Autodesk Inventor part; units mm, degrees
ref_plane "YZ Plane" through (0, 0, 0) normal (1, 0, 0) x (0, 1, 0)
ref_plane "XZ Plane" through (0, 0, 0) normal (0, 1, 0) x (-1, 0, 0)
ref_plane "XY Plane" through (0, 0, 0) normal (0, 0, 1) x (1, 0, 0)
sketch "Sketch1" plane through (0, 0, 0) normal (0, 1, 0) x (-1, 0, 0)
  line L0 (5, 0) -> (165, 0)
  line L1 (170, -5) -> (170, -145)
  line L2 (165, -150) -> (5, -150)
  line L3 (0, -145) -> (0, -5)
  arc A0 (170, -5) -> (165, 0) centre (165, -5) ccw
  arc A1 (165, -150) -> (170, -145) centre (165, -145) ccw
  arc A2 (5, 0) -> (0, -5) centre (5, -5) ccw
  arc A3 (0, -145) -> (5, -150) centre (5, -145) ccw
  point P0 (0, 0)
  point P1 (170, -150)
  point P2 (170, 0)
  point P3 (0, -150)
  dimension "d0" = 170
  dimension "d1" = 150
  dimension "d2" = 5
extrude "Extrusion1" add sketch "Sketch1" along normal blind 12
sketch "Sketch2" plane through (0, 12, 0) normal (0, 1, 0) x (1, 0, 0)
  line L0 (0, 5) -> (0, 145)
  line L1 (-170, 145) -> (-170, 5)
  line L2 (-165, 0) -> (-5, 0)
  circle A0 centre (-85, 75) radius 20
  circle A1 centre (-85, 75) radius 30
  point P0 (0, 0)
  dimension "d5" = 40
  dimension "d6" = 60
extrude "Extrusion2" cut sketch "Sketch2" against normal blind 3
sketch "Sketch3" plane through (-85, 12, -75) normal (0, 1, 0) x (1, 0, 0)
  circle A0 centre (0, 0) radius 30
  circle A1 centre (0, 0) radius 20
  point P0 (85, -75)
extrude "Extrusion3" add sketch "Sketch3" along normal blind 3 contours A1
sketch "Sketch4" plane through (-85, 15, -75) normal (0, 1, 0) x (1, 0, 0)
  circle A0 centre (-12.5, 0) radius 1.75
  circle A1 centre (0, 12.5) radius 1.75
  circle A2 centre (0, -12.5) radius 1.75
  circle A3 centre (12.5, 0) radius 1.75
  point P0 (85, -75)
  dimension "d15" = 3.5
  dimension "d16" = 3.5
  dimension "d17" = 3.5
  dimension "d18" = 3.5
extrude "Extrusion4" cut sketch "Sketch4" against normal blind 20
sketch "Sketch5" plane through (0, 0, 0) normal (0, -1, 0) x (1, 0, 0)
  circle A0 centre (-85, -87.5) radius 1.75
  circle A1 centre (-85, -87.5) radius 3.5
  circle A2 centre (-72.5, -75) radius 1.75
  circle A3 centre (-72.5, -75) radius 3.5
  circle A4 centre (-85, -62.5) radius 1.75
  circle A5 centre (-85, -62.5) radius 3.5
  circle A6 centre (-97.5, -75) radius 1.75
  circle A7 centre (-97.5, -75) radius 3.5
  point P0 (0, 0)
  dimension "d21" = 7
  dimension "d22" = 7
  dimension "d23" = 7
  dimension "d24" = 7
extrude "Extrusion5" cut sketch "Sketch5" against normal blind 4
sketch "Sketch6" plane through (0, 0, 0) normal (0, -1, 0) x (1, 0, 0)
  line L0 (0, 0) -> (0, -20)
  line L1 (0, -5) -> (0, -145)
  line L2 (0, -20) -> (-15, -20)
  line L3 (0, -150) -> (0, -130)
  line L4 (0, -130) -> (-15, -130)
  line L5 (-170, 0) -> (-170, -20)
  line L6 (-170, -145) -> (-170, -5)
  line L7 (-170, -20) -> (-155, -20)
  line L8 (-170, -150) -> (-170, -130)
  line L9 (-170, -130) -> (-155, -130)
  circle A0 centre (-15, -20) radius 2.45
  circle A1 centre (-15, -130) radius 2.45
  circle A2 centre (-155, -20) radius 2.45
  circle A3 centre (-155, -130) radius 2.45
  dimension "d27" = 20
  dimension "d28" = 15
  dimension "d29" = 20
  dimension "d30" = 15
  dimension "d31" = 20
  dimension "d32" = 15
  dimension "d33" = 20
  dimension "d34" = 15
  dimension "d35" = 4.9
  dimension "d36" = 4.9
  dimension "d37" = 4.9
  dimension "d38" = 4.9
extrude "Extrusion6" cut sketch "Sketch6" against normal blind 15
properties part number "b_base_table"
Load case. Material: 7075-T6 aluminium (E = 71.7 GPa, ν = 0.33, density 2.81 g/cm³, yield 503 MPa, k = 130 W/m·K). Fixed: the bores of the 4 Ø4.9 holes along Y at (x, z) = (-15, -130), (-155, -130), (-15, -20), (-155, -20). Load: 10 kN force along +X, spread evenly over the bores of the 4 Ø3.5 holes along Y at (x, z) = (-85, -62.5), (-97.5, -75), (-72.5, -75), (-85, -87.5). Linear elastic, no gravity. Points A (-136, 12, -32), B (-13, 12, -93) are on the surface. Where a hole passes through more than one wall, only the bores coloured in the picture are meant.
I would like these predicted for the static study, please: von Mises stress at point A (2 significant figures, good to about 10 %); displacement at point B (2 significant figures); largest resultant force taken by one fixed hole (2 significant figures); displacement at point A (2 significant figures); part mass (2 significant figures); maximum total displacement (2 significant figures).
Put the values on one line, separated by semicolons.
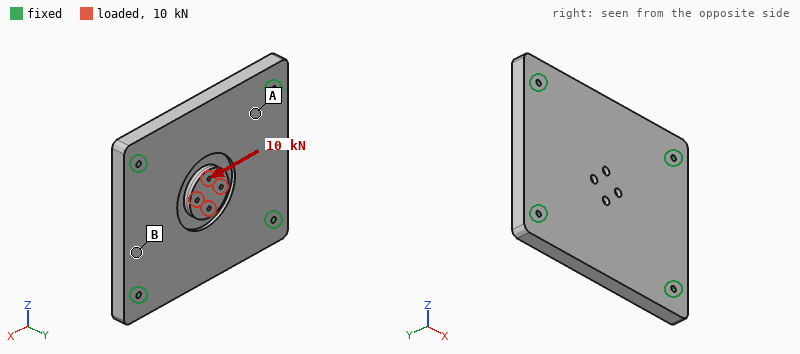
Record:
6.3 MPa; 5.5 µm; 2.7 kN; 3.5 µm; 850 g; 19 µm
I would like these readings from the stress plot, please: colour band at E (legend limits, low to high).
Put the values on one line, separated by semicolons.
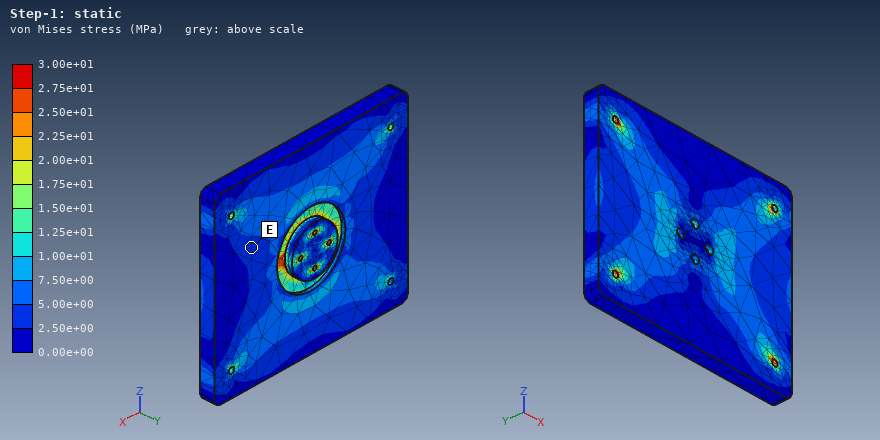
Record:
2.50e+00 to 5.00e+00 MPa
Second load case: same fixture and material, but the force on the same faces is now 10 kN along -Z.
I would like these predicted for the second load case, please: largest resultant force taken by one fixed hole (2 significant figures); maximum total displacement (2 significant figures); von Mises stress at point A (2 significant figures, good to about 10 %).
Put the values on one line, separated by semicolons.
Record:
2.8 kN; 22 µm; 7.2 MPa
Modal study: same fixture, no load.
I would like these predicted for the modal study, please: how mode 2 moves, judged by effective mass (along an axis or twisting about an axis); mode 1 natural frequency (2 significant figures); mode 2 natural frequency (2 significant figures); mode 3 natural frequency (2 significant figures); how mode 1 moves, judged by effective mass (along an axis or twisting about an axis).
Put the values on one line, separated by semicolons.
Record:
twisting about X; 2100 Hz; 3100 Hz; 3900 Hz; along Y
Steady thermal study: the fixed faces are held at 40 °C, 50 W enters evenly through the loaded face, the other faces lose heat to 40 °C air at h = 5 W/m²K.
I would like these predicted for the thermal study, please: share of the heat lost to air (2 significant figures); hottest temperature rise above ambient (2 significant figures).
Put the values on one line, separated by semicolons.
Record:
3.5 %; 17 K
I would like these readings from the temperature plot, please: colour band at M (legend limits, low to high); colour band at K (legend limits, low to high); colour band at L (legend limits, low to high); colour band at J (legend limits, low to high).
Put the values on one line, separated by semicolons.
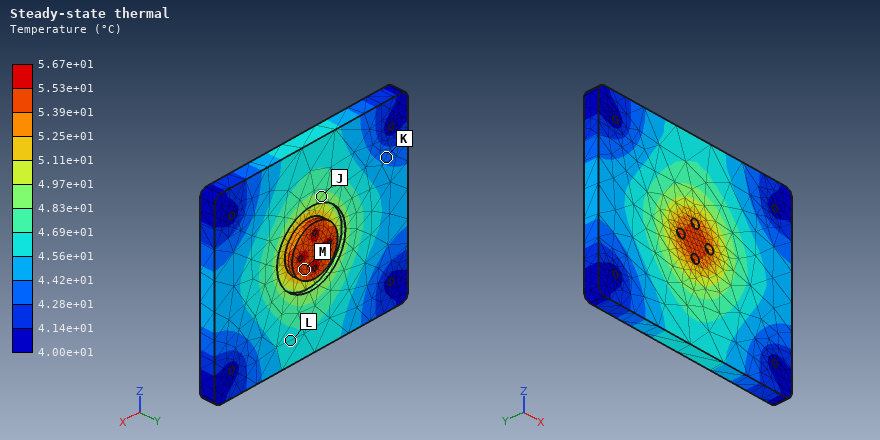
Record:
5.39e+01 to 5.53e+01 °C; 4.28e+01 to 4.42e+01 °C; 4.56e+01 to 4.69e+01 °C; 4.83e+01 to 4.97e+01 °C
